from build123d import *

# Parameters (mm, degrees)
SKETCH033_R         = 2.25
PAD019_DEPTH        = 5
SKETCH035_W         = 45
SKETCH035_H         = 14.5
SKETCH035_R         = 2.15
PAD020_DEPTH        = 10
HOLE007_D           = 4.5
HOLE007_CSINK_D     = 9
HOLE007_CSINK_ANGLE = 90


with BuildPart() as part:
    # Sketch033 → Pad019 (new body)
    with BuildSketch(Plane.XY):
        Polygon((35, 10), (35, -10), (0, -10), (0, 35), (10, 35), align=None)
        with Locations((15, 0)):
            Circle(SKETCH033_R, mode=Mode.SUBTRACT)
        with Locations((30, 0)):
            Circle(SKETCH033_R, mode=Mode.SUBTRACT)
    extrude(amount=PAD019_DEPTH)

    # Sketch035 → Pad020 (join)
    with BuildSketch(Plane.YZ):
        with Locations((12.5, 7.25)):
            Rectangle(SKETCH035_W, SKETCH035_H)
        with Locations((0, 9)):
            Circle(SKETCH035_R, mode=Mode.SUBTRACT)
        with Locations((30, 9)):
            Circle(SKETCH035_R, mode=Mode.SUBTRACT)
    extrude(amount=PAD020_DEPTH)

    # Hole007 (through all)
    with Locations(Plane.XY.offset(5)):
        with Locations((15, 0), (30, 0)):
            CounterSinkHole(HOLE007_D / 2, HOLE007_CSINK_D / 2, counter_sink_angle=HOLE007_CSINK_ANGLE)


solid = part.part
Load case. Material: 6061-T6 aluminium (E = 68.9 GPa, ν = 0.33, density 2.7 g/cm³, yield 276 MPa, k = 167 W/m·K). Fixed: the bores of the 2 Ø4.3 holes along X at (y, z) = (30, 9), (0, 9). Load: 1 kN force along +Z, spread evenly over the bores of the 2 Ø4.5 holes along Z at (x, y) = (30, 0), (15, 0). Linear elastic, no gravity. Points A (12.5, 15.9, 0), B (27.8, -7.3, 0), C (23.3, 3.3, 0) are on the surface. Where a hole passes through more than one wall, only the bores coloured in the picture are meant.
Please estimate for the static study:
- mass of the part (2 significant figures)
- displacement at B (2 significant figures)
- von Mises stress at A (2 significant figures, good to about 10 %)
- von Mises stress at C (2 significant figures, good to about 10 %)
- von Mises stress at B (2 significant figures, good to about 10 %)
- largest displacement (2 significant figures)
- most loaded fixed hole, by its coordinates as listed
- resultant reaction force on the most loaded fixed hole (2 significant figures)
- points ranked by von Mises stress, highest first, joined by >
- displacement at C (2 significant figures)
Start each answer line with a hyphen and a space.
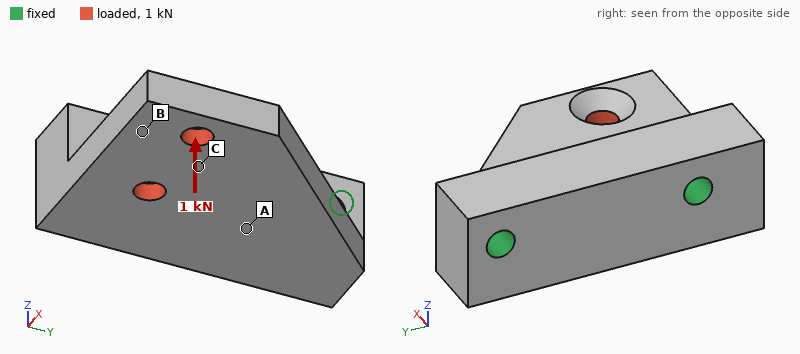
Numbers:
- 27 g
- 0.12 mm
- 53 MPa
- 40 MPa
- 12 MPa
- 0.18 mm
- (0, 9)
- 990 N
- A > C > B
- 0.078 mm
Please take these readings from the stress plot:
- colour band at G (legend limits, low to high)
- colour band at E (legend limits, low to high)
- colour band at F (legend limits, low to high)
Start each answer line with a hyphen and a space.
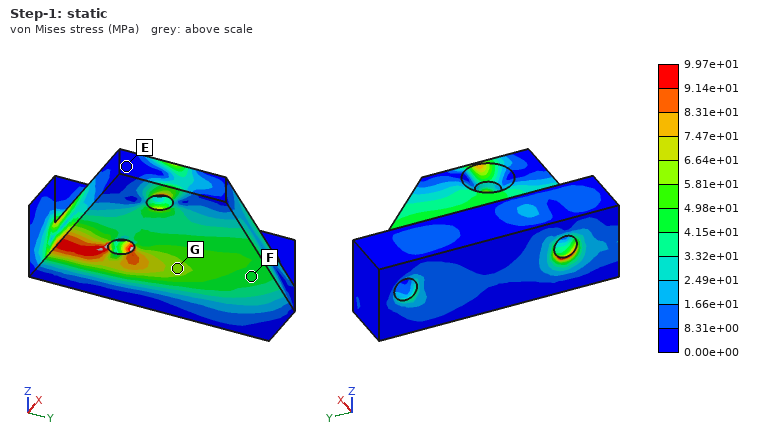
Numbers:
- 5.81e+01 to 6.64e+01 MPa
- 0.00e+00 to 8.31e+00 MPa
- 4.15e+01 to 4.98e+01 MPa
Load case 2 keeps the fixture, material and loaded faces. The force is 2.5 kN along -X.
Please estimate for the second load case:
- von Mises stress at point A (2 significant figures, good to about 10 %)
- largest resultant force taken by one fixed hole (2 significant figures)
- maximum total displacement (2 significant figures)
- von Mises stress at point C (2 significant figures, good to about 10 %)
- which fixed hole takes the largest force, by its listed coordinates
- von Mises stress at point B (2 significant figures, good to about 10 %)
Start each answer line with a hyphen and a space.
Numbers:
- 18 MPa
- 2.3 kN
- 67 µm
- 32 MPa
- (0, 9)
- 17 MPa
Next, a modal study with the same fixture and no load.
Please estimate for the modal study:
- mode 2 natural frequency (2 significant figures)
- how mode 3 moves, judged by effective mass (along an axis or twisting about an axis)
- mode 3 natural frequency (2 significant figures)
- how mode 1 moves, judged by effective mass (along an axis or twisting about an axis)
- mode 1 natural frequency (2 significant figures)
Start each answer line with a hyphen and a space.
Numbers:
- 13 kHz
- along Y
- 19 kHz
- along Z
- 5700 Hz
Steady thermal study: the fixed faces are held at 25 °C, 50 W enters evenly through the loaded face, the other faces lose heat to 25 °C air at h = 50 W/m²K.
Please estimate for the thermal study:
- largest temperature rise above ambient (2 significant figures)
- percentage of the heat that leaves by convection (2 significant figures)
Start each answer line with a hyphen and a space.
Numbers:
- 49 K
- 5.5 %
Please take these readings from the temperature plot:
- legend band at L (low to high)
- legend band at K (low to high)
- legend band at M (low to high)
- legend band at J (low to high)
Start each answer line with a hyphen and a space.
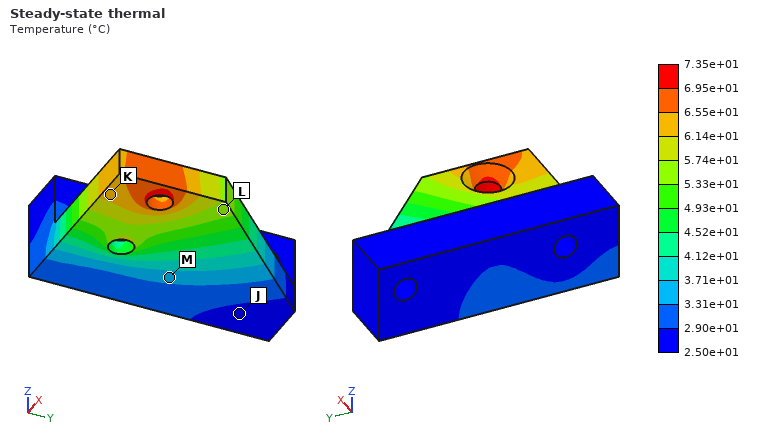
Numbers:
- 5.33e+01 to 5.74e+01 °C
- 6.14e+01 to 6.55e+01 °C
- 3.31e+01 to 3.71e+01 °C
- 2.50e+01 to 2.90e+01 °C
